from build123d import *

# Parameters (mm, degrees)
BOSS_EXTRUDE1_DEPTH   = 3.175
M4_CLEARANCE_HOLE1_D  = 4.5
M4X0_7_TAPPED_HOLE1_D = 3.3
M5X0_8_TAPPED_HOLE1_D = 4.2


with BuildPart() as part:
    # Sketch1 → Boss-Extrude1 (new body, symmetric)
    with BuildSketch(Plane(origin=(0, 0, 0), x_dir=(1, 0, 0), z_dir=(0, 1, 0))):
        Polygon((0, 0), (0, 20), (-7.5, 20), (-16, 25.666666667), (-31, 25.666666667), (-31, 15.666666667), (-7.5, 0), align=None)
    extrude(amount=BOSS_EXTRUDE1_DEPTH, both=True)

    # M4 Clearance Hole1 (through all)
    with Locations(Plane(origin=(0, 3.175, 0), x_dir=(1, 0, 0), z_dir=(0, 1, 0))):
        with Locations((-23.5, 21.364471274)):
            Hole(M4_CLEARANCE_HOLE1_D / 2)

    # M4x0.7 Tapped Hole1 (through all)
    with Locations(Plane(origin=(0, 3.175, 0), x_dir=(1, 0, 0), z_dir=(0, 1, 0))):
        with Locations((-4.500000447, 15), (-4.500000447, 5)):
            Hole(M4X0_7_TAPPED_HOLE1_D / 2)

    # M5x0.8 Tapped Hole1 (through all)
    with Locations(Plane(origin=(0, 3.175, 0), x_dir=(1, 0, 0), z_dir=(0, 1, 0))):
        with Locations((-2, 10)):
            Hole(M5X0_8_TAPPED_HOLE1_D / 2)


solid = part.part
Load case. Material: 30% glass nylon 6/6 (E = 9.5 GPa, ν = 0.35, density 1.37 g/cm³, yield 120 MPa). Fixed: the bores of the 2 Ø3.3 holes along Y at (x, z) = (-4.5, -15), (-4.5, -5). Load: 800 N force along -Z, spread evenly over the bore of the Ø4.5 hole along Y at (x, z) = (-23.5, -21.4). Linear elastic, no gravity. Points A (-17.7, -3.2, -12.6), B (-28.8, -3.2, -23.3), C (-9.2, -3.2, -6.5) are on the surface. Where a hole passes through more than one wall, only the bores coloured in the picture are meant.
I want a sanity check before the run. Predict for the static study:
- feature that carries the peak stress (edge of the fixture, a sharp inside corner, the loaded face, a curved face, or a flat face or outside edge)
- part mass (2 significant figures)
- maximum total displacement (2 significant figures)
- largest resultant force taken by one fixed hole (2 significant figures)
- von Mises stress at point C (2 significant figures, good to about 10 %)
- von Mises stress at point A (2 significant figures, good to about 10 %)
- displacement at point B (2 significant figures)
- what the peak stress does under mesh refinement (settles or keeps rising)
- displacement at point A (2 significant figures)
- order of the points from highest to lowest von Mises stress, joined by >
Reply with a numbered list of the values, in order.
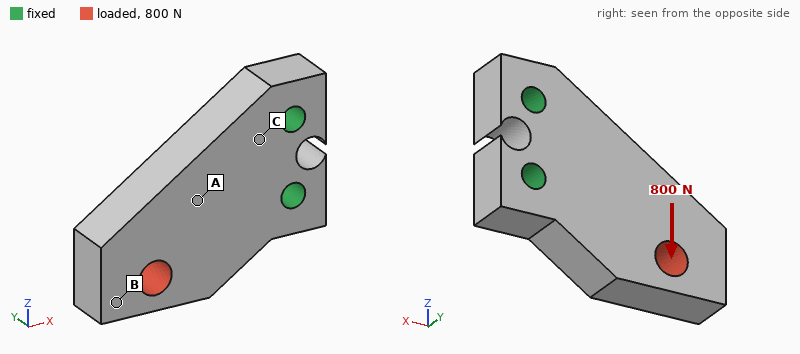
1. edge of the fixture
2. 4.3 g
3. 0.20 mm
4. 1.3 kN
5. 29 MPa
6. 18 MPa
7. 0.18 mm
8. keeps rising
9. 0.067 mm
10. C > A > B
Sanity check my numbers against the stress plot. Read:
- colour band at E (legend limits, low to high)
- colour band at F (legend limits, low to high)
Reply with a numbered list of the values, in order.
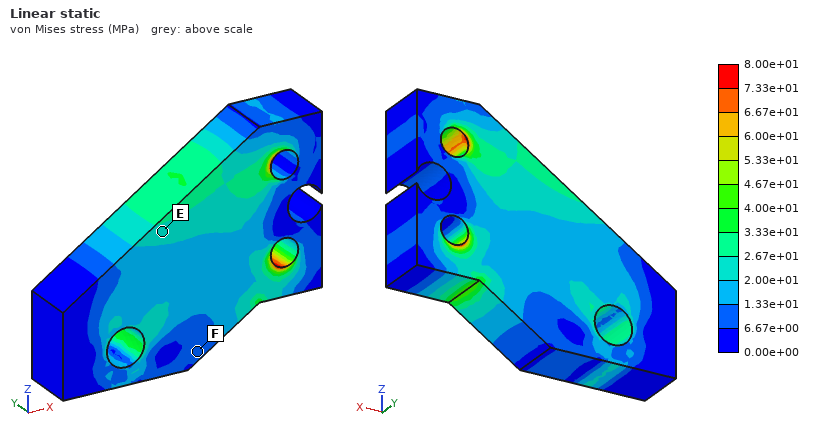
1. 2.00e+01 to 2.67e+01 MPa
2. 6.67e+00 to 1.33e+01 MPa
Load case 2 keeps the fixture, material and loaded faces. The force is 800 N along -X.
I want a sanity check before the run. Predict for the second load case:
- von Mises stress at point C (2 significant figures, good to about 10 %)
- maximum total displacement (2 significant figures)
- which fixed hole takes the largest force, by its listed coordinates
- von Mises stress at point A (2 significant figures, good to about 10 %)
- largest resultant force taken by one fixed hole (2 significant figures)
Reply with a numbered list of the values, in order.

1. 9.1 MPa
2. 0.13 mm
3. (-4.5, -15)
4. 7.0 MPa
5. 1.1 kN
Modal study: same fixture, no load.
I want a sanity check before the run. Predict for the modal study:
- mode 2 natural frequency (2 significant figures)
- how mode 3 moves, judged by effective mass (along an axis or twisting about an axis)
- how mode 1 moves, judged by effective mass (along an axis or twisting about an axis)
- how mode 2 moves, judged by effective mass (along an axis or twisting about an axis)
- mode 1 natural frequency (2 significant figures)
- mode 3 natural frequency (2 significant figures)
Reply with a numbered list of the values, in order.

1. 8600 Hz
2. twisting about X
3. along Y
4. along Z
5. 4200 Hz
6. 12 kHz
